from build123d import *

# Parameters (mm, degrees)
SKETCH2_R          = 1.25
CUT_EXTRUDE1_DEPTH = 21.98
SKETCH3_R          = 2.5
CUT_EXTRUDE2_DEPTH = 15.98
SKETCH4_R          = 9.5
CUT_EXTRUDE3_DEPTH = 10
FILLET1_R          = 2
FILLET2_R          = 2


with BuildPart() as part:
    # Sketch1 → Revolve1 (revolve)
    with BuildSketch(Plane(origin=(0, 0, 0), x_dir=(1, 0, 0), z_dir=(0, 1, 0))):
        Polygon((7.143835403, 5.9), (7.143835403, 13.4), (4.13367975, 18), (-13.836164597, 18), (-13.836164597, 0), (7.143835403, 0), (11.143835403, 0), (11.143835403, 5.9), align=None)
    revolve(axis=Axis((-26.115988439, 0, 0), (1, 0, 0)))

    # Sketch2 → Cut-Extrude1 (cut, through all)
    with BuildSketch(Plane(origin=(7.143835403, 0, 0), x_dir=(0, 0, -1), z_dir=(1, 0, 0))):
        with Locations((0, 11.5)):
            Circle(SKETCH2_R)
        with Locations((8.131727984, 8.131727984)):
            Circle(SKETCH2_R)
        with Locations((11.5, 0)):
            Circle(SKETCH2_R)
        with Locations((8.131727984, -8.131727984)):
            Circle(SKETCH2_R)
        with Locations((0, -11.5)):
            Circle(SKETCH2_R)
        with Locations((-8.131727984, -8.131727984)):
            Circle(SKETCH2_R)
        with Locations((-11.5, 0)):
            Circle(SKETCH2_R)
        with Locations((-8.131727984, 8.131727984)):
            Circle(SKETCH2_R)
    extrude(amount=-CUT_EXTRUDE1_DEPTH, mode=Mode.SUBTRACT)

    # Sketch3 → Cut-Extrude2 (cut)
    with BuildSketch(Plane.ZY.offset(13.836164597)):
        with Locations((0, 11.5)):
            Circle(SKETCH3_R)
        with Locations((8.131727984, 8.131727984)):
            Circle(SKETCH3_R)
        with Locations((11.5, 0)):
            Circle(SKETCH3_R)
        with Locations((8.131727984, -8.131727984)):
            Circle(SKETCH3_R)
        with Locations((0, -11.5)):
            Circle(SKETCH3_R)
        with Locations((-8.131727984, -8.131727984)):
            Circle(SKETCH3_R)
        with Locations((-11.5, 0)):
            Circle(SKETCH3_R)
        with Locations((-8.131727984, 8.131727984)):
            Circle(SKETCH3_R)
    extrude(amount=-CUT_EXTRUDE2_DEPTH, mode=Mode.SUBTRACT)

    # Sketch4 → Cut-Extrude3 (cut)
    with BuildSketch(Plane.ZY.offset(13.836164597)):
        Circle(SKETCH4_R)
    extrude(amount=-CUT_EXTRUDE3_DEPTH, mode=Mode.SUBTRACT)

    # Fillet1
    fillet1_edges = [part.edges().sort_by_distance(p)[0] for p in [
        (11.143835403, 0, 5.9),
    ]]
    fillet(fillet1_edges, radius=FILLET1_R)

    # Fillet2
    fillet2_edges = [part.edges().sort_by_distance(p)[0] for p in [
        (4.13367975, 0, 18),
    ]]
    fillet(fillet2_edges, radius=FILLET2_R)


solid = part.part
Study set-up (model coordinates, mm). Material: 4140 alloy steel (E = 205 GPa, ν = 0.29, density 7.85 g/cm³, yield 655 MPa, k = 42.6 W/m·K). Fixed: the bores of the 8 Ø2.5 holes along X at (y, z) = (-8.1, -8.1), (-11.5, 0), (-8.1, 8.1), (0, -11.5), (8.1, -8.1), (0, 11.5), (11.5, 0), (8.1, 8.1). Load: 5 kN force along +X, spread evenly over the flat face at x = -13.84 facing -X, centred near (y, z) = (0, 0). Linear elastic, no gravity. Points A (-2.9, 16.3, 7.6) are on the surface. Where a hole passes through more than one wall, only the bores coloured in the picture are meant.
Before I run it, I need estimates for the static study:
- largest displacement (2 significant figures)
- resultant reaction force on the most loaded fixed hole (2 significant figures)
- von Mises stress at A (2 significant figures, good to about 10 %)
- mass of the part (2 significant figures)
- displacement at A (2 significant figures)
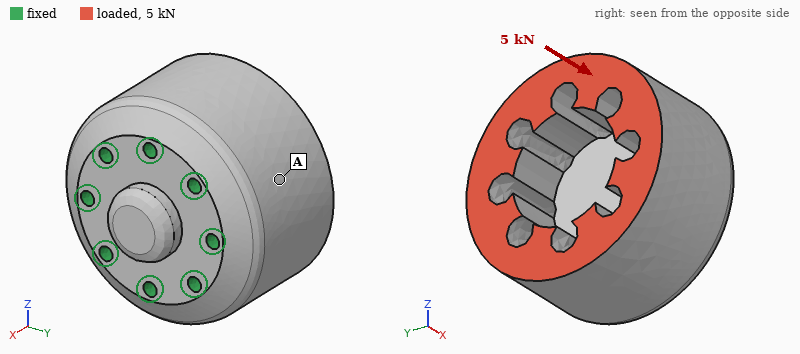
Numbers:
1.3 µm
630 N
6.2 MPa
120 g
0.88 µm
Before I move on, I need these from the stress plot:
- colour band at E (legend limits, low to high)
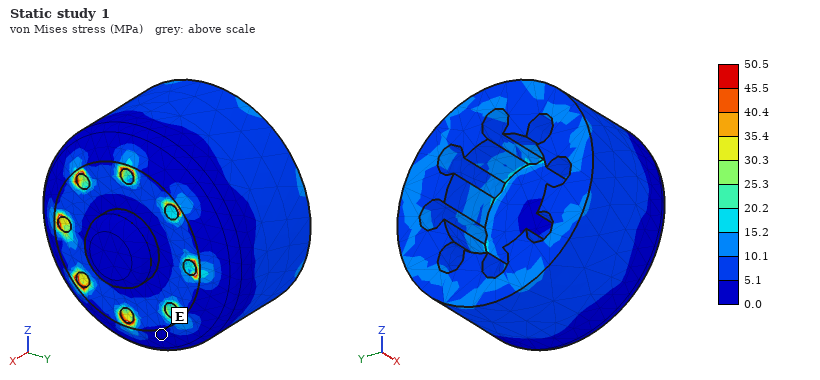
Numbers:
0.0 to 5.1 MPa
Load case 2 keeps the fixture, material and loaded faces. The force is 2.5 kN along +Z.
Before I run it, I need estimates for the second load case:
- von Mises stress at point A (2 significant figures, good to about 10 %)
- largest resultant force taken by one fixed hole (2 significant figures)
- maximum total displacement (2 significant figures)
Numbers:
9.7 MPa
850 N
5.1 µm
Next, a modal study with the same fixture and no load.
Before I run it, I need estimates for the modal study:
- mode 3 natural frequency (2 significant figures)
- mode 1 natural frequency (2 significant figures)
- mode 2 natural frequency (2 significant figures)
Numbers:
25 kHz
23 kHz
23 kHz
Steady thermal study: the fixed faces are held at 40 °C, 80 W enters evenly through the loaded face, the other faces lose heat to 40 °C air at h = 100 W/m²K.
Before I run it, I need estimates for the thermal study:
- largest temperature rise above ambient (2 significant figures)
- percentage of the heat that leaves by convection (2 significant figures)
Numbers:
55 K
17 %
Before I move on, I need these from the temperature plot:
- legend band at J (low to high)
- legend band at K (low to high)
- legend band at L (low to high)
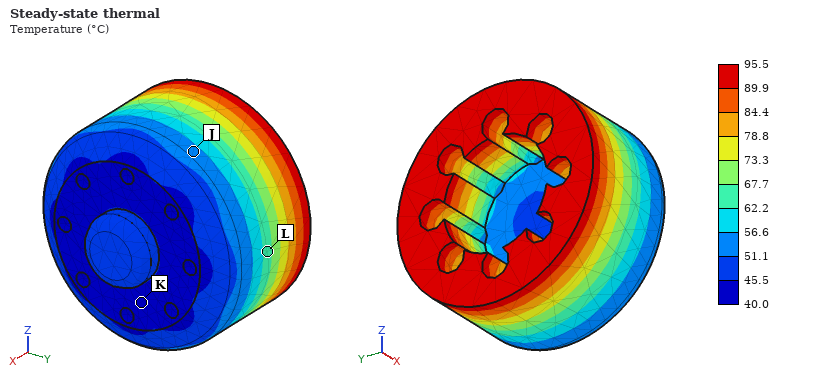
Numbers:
51.1 to 56.6 °C
40.0 to 45.5 °C
62.2 to 67.7 °C
